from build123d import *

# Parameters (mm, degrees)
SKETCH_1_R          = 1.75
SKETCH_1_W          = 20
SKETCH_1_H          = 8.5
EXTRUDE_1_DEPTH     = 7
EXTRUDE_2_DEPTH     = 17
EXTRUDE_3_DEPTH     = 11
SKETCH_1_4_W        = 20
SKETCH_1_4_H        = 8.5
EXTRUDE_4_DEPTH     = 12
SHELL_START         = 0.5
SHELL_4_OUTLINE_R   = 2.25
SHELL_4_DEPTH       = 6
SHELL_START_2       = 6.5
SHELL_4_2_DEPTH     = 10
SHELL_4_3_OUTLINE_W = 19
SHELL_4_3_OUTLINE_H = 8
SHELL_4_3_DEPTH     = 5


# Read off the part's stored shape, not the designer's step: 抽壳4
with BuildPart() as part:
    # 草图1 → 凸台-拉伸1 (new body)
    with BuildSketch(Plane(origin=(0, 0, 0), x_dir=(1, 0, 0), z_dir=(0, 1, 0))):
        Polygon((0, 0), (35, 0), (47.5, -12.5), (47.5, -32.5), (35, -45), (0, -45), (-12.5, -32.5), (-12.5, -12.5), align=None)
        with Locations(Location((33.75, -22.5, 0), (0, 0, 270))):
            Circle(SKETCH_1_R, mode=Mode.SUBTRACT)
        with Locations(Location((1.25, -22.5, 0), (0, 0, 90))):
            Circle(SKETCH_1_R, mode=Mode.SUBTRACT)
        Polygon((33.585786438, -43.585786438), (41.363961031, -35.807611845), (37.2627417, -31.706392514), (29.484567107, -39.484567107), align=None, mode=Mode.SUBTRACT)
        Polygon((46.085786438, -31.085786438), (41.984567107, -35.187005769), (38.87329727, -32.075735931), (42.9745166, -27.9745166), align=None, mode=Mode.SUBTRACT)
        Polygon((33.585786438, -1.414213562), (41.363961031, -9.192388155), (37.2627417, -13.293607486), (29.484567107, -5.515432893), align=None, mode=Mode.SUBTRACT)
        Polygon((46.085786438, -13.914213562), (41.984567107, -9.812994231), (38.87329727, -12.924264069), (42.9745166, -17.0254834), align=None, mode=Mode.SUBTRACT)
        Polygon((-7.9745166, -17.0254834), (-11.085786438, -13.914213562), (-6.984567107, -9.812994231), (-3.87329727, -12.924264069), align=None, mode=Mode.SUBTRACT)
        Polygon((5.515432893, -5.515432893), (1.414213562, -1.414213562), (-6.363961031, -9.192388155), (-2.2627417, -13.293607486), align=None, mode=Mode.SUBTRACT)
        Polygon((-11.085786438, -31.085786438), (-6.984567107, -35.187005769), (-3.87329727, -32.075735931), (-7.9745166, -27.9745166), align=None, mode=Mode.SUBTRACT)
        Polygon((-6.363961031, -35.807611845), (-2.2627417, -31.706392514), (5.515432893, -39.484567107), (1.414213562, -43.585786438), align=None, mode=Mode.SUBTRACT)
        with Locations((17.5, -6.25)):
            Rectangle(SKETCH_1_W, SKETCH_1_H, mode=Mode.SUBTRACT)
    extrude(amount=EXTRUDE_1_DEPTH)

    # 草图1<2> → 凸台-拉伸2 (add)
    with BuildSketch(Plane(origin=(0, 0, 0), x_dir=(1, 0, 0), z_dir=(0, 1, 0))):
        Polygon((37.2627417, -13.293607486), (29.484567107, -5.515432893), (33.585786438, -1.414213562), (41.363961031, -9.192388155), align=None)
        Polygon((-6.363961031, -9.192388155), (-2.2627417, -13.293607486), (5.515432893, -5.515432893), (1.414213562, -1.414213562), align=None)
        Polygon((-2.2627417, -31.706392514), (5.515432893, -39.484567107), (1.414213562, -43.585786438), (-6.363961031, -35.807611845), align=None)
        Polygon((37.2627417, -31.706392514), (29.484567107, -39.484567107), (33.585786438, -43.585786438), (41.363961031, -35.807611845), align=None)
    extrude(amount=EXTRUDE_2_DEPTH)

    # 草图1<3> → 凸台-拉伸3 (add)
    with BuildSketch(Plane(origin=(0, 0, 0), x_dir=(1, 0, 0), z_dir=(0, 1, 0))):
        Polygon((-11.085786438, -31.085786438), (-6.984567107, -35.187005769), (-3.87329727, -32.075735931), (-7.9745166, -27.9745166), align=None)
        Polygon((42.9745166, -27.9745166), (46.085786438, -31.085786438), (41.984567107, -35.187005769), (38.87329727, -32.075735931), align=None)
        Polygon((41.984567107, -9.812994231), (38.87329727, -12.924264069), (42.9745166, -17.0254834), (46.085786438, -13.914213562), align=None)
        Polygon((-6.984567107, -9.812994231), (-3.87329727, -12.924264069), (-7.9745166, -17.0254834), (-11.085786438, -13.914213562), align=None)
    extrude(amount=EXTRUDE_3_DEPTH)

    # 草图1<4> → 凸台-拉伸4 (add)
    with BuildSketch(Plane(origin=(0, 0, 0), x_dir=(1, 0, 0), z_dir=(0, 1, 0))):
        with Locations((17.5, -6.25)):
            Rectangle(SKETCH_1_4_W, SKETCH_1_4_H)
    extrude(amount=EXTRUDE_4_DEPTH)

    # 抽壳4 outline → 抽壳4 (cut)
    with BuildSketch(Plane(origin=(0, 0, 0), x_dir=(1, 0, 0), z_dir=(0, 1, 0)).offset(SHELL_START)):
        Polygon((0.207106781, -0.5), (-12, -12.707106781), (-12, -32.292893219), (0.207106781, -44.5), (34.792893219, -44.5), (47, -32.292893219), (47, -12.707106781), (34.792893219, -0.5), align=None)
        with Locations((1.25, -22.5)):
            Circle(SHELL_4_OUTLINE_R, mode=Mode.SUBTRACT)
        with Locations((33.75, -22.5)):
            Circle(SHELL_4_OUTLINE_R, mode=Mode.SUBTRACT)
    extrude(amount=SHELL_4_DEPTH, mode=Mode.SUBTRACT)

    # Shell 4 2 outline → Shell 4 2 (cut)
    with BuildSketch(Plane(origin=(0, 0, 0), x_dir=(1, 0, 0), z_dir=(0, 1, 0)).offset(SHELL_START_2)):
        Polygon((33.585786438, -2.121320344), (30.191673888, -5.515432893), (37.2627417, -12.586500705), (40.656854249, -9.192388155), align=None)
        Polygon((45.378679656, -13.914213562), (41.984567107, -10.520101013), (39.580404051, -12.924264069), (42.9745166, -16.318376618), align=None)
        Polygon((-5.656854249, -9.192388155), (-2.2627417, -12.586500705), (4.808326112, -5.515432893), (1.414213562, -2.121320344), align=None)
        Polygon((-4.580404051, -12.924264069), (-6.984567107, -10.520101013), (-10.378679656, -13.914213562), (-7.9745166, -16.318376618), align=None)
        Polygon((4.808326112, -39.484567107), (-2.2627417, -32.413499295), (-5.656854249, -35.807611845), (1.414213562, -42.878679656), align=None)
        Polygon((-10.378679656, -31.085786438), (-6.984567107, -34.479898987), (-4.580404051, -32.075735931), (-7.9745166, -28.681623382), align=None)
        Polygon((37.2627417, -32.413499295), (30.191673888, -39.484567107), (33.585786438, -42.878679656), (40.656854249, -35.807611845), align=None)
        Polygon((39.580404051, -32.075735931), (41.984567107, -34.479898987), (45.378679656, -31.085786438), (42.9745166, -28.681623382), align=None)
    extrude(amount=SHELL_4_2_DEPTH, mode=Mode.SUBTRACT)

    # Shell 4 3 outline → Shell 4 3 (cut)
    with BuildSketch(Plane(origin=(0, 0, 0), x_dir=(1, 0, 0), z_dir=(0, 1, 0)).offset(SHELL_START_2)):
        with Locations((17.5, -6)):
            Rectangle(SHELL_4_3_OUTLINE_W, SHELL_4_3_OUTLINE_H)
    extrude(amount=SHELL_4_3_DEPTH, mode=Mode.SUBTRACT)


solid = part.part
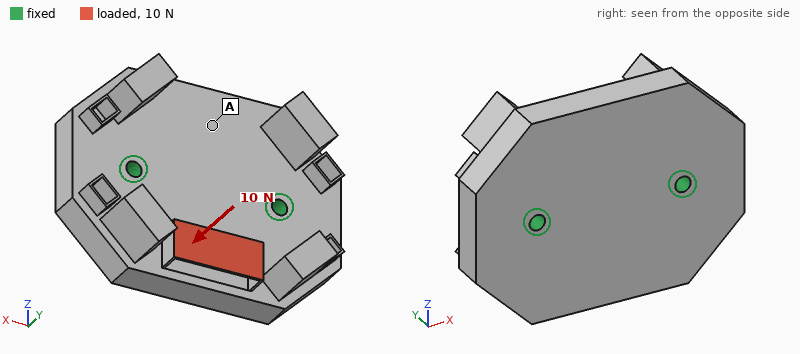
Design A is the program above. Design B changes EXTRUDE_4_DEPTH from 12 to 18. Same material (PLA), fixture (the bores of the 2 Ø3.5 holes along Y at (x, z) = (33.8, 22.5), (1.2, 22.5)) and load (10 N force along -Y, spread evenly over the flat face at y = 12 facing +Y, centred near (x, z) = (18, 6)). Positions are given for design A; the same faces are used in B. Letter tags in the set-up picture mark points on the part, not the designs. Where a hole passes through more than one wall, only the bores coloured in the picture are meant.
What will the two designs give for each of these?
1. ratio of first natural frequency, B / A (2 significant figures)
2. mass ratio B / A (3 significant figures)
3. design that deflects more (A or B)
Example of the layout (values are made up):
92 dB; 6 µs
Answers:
0.81; 1.27; A
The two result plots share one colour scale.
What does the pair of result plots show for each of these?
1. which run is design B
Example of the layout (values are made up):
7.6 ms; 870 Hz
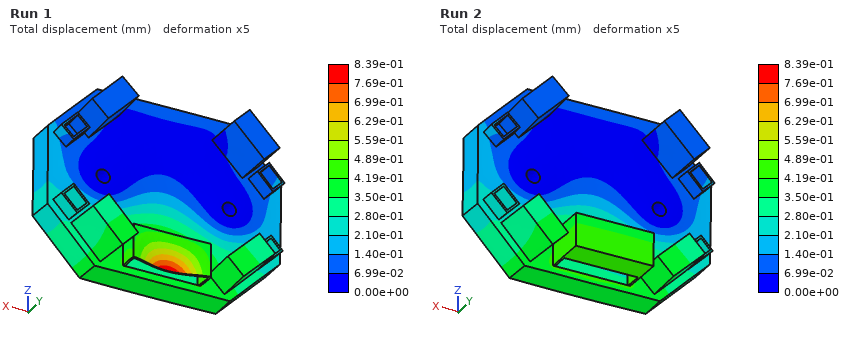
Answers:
Run 2
